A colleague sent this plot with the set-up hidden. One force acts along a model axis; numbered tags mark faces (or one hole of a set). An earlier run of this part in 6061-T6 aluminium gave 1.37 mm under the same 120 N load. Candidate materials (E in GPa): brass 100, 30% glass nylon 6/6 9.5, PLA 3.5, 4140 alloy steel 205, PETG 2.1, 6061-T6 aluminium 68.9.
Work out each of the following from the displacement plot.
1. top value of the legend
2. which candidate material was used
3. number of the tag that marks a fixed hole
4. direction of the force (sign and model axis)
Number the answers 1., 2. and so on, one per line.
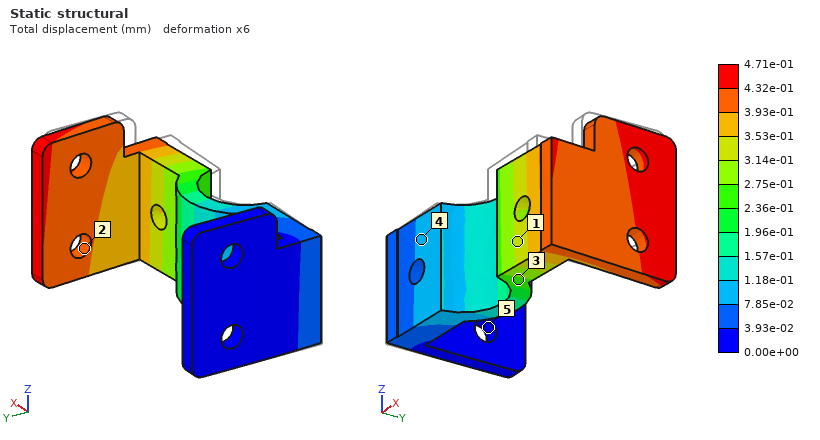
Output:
1. 4.71e-01 mm
2. 4140 alloy steel
3. 5
4. +Y
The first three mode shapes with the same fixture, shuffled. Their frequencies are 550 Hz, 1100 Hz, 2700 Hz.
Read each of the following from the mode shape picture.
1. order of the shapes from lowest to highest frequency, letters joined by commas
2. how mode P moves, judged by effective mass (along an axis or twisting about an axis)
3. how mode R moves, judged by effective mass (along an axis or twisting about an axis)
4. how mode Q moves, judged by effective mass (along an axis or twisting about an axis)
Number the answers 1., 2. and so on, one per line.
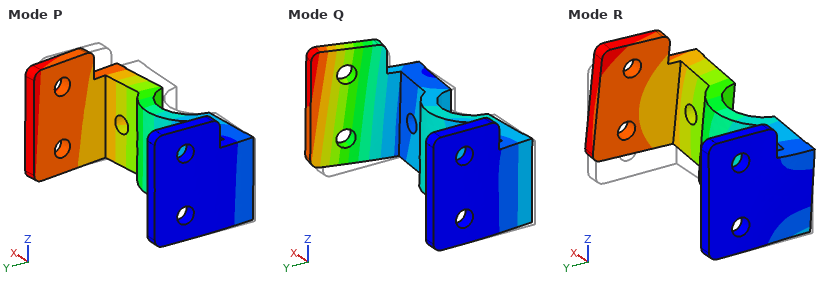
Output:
1. P, R, Q
2. along Y
3. along Z
4. along X
